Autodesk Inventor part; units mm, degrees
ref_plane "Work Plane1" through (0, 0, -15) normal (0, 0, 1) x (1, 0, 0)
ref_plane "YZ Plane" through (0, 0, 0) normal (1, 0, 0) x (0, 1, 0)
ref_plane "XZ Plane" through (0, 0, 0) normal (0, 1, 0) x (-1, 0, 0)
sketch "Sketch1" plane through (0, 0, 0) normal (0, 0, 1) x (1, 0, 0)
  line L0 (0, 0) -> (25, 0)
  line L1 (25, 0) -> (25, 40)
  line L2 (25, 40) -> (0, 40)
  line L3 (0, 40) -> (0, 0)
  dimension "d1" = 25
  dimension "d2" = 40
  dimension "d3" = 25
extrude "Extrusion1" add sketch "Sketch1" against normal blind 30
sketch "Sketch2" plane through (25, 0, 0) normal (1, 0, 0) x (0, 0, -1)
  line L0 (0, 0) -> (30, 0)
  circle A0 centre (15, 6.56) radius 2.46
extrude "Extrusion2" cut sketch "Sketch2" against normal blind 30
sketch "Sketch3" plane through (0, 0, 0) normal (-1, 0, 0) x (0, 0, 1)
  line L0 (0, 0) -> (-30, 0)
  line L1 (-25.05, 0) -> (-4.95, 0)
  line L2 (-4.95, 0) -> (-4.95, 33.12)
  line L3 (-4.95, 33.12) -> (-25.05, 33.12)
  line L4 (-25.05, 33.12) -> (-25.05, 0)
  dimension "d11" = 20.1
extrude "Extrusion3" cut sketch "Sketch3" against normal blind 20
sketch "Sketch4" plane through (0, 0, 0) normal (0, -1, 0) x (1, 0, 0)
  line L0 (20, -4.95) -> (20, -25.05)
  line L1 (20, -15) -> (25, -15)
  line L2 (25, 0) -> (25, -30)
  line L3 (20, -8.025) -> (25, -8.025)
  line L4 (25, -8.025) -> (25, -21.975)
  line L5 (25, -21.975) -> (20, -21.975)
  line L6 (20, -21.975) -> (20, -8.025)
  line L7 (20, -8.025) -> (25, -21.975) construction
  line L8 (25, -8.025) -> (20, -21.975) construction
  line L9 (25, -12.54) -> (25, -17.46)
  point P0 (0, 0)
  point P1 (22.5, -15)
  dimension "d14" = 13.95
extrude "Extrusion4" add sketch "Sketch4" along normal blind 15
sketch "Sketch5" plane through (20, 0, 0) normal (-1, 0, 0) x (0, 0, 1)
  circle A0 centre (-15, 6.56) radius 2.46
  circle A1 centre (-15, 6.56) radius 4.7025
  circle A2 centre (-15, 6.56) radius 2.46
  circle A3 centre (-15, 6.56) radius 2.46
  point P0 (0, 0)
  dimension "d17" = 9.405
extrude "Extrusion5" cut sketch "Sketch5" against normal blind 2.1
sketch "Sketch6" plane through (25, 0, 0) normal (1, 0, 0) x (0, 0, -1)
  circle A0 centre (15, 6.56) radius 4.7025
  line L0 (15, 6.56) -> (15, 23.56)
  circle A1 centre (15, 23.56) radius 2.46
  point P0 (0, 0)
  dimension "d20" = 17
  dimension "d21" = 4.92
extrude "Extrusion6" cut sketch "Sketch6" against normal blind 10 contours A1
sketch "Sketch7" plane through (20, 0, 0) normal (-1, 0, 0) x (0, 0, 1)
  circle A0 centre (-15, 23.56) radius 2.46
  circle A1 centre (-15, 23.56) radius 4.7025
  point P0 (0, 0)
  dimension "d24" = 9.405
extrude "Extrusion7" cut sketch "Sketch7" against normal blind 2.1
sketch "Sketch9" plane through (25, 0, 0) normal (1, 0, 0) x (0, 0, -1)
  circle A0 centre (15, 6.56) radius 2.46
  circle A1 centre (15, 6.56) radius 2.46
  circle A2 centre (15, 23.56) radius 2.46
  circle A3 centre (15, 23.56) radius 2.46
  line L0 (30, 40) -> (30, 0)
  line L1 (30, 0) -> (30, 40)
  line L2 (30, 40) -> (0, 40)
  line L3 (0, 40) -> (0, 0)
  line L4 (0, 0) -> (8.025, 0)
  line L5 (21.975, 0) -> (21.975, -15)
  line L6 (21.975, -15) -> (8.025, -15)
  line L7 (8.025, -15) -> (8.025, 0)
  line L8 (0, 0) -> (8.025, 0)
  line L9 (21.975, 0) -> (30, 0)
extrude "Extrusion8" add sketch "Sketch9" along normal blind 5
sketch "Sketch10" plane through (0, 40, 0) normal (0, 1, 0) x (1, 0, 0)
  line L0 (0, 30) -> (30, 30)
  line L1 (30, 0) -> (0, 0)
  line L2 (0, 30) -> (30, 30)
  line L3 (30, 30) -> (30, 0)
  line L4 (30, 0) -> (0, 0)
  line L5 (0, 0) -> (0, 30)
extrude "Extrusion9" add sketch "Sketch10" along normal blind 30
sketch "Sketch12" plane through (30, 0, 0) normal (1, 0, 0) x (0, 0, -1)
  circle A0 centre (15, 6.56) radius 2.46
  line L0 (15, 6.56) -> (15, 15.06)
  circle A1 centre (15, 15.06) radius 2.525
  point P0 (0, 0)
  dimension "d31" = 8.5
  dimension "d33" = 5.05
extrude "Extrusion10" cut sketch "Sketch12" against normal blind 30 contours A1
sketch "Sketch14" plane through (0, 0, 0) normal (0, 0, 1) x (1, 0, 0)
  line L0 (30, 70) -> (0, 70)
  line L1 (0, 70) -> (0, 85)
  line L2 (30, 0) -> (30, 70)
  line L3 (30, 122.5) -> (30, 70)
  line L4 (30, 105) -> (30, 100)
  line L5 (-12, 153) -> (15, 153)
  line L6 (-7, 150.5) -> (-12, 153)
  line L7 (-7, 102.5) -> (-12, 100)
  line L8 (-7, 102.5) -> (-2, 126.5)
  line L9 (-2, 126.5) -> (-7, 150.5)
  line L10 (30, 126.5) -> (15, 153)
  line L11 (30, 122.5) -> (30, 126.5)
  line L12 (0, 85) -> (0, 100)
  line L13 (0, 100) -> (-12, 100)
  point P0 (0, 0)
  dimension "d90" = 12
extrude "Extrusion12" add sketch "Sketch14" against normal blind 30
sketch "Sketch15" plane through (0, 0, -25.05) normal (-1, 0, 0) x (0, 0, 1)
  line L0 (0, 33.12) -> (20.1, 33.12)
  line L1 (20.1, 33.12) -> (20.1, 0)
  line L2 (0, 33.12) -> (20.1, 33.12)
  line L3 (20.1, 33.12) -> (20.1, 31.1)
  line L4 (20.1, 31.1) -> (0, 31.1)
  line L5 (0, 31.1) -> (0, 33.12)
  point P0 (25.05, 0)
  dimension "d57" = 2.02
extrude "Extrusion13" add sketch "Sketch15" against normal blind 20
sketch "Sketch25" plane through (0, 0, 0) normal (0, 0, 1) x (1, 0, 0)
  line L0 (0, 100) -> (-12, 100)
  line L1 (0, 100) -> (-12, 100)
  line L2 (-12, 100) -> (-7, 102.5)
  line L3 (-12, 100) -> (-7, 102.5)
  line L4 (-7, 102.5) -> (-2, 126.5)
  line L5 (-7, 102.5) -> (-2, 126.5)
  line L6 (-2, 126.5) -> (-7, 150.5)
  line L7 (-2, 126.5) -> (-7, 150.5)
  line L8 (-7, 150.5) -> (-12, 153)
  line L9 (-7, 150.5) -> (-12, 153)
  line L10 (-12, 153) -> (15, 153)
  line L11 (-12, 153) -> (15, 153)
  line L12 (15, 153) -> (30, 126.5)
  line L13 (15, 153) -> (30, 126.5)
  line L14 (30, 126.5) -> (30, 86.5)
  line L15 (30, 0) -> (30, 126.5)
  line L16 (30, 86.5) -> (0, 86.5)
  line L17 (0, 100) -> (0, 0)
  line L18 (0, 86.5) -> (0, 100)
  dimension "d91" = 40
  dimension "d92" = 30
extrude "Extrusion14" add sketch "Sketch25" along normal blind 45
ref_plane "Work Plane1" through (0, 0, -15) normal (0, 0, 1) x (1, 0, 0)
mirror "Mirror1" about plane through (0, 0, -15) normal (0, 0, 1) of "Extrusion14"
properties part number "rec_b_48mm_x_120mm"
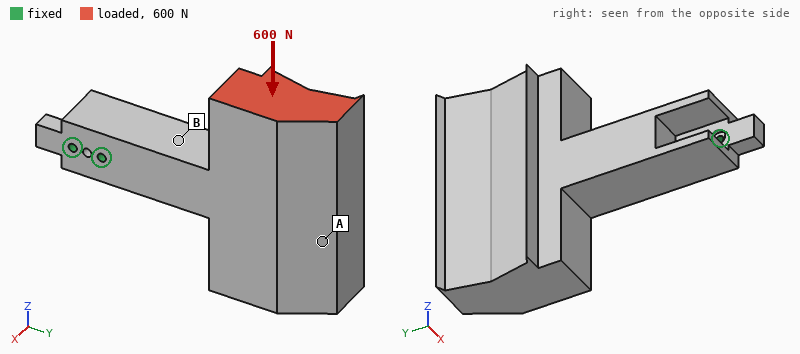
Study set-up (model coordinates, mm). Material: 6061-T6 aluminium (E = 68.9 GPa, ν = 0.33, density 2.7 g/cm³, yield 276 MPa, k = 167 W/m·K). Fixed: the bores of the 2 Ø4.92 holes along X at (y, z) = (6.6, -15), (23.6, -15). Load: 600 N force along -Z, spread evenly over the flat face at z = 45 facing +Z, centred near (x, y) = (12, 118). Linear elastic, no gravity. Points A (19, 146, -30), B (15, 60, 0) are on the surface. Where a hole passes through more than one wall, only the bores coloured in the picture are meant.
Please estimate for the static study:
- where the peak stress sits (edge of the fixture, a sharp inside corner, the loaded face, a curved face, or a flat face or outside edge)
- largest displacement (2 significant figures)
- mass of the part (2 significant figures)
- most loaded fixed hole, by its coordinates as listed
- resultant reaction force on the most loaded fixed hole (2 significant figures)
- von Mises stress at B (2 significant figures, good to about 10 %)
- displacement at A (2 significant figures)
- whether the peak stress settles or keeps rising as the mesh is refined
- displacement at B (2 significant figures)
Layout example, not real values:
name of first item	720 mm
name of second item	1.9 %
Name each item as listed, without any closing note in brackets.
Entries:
where the peak stress sits	edge of the fixture
largest displacement	0.18 mm
mass of the part	850 g
most loaded fixed hole, by its coordinates as listed	(23.6, -15)
resultant reaction force on the most loaded fixed hole	3.0 kN
von Mises stress at B	7.8 MPa
displacement at A	0.15 mm
whether the peak stress settles or keeps rising as the mesh is refined	keeps rising
displacement at B	0.041 mm
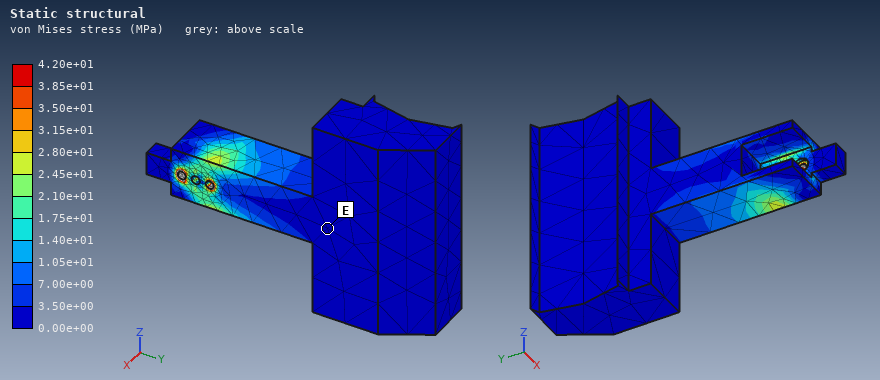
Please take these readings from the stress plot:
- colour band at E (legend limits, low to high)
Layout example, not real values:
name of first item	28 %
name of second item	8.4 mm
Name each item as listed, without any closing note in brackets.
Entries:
colour band at E	0.00e+00 to 3.50e+00 MPa
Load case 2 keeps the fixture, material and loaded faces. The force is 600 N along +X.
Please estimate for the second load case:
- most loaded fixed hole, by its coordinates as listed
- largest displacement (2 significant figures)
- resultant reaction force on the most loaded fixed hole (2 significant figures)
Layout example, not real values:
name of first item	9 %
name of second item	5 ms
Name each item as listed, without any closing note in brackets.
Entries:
most loaded fixed hole, by its coordinates as listed	(23.6, -15)
largest displacement	0.37 mm
resultant reaction force on the most loaded fixed hole	2.9 kN
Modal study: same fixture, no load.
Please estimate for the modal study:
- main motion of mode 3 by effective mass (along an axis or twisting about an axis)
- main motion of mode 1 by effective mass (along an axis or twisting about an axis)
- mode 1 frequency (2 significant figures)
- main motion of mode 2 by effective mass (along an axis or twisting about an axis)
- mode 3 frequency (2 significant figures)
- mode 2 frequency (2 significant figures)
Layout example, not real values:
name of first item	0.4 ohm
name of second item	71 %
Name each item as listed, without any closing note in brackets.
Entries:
main motion of mode 3 by effective mass	twisting about Y
main motion of mode 1 by effective mass	along X
mode 1 frequency	370 Hz
main motion of mode 2 by effective mass	along Z
mode 3 frequency	650 Hz
mode 2 frequency	400 Hz
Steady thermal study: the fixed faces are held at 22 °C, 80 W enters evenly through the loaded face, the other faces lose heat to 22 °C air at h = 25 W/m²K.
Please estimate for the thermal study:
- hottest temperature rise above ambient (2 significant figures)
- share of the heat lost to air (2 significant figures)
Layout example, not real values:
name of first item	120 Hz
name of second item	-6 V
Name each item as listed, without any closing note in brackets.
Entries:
hottest temperature rise above ambient	48 K
share of the heat lost to air	37 %
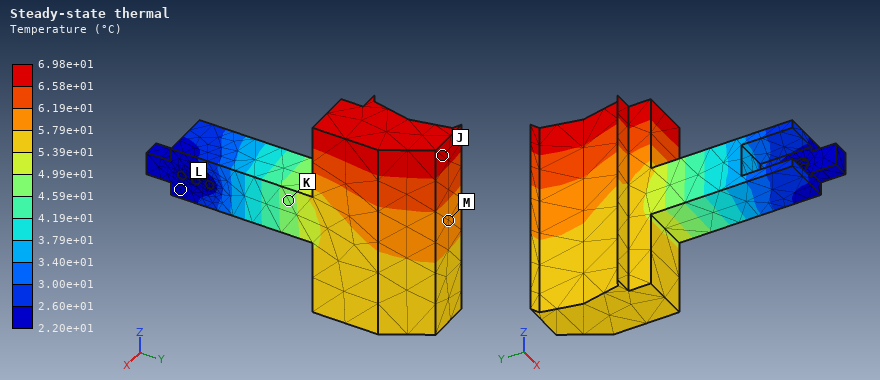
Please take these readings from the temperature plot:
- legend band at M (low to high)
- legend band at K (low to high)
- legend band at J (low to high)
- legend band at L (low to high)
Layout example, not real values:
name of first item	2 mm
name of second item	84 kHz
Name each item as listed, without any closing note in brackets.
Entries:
legend band at M	5.79e+01 to 6.19e+01 °C
legend band at K	4.59e+01 to 4.99e+01 °C
legend band at J	6.58e+01 to 6.98e+01 °C
legend band at L	2.20e+01 to 2.60e+01 °C
